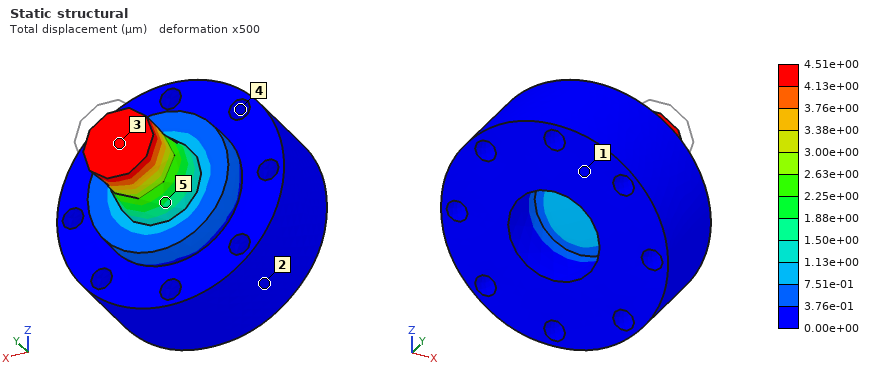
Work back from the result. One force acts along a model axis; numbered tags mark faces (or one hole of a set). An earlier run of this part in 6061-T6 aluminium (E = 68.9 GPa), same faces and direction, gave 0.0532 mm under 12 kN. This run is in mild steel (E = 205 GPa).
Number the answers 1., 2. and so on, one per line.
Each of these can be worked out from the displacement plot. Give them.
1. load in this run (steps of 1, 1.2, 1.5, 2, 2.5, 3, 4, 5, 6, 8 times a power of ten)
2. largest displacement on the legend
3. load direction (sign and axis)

1. 3 kN
2. 4.51e+00 µm
3. -Y
